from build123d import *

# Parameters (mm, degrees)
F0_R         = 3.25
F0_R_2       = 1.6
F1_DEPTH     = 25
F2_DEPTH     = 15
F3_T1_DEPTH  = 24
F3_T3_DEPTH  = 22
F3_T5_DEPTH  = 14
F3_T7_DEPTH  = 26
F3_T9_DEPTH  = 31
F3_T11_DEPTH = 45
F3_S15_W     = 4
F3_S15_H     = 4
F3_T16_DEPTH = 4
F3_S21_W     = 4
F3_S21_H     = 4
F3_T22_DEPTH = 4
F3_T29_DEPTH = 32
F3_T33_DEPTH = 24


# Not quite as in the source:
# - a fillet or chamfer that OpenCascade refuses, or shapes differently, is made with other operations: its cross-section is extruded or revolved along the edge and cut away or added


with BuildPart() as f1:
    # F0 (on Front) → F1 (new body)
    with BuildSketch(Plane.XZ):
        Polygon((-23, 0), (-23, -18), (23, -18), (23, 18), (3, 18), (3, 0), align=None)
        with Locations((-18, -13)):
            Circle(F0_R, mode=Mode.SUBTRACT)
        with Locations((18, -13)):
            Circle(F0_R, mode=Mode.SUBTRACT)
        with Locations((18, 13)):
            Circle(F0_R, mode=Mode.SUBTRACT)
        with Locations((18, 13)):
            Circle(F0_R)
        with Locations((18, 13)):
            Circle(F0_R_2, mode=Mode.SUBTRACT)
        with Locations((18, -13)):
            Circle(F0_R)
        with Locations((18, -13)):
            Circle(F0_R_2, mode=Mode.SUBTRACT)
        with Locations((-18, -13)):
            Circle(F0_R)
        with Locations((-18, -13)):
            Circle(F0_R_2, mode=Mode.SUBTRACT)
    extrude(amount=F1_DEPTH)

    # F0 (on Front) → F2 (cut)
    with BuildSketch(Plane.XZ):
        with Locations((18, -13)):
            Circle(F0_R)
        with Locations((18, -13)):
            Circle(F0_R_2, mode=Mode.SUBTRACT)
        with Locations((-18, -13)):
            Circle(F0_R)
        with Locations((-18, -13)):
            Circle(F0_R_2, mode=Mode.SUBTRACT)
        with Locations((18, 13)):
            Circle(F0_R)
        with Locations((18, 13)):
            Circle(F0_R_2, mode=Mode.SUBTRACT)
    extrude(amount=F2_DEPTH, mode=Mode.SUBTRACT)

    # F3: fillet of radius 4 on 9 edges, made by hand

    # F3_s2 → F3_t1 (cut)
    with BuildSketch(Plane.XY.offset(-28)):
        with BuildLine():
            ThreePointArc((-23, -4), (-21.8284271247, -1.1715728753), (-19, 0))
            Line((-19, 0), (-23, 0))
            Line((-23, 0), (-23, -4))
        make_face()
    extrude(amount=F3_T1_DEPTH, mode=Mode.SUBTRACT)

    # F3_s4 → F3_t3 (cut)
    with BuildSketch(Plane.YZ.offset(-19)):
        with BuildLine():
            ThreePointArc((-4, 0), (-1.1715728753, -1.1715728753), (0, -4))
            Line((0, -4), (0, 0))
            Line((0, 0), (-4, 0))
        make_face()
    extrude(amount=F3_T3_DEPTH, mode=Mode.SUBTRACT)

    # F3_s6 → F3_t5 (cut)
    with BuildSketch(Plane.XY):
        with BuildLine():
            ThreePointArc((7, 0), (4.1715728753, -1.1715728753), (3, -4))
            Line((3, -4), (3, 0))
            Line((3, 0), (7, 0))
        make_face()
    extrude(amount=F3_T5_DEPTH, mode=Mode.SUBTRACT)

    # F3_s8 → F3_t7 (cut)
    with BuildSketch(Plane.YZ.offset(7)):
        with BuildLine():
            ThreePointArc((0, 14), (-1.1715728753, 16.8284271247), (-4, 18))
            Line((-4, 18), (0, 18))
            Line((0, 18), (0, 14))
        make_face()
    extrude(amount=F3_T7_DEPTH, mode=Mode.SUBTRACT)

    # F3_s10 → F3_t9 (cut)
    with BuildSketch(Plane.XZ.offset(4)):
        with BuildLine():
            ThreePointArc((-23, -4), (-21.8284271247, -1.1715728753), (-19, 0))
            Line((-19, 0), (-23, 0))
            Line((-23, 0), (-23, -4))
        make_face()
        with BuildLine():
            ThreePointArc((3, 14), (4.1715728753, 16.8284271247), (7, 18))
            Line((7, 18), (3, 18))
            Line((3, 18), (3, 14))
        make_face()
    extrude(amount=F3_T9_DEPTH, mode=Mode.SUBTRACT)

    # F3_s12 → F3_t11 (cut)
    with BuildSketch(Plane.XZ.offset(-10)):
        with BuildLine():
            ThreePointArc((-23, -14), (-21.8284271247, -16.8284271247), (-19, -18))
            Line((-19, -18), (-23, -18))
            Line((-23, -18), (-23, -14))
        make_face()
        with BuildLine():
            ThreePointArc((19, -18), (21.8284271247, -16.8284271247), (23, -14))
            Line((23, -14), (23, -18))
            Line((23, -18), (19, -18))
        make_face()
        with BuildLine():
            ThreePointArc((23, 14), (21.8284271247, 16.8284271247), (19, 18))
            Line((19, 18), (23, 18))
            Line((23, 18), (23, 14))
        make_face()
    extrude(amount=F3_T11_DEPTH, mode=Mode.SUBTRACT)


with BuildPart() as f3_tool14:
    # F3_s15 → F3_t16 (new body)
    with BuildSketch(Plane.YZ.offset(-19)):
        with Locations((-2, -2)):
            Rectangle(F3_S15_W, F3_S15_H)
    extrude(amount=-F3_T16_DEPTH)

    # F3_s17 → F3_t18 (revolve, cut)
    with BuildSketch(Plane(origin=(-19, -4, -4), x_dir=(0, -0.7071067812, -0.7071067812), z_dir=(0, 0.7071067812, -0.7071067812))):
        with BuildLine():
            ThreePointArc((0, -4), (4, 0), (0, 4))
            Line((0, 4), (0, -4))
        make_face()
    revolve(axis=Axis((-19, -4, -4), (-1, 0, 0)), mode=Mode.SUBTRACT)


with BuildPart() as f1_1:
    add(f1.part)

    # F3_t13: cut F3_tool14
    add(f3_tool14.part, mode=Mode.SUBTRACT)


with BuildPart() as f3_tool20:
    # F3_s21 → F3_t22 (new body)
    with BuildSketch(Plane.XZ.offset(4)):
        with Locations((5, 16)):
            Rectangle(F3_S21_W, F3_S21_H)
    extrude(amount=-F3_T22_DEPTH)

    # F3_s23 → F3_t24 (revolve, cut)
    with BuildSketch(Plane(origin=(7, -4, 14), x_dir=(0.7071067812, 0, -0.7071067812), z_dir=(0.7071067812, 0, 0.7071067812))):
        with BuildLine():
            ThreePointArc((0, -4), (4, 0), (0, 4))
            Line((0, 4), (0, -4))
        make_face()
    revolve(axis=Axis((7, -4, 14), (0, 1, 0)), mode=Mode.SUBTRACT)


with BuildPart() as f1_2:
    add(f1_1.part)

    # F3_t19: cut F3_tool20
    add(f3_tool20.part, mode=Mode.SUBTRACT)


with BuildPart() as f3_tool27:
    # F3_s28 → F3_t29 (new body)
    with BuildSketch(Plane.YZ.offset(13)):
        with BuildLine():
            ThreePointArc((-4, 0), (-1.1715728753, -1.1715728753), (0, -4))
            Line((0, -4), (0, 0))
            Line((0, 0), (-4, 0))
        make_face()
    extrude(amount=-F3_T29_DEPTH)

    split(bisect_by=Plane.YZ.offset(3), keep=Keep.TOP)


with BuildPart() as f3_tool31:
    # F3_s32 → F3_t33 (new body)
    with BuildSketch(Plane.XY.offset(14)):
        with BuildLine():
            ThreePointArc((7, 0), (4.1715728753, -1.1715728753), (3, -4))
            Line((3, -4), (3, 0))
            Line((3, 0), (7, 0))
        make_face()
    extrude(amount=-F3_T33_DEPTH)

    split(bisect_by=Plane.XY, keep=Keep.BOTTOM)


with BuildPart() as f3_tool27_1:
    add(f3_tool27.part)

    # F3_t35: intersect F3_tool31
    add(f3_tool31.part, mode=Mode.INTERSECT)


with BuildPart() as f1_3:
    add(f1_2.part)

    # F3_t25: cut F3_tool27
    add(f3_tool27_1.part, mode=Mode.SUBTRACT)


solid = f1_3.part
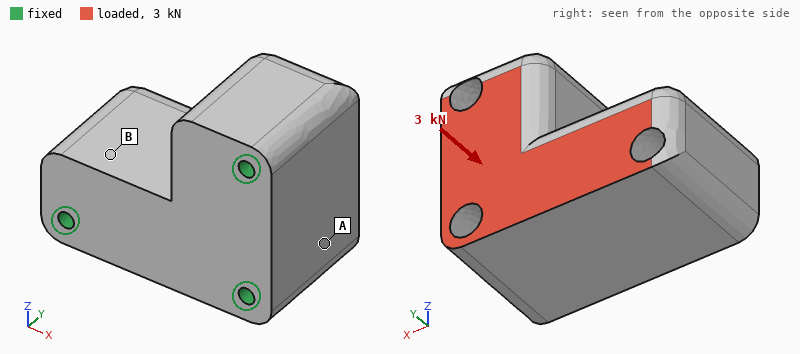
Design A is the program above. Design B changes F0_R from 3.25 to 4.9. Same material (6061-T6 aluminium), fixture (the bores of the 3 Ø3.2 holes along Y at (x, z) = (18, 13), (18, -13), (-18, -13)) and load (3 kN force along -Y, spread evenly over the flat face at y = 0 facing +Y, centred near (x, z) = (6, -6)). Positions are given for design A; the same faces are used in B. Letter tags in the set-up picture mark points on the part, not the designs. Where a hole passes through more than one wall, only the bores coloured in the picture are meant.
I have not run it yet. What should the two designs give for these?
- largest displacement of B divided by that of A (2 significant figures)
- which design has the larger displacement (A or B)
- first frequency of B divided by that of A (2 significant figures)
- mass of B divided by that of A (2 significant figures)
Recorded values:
1.3
B
0.94
0.93
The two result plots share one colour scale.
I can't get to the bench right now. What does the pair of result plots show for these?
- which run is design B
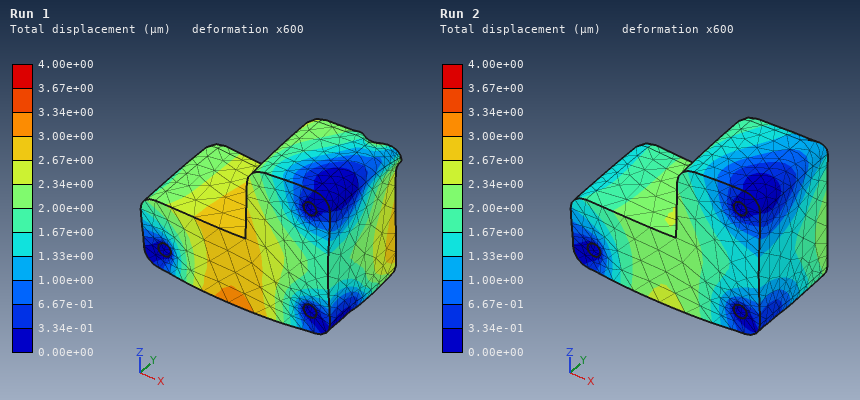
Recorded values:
Run 1
